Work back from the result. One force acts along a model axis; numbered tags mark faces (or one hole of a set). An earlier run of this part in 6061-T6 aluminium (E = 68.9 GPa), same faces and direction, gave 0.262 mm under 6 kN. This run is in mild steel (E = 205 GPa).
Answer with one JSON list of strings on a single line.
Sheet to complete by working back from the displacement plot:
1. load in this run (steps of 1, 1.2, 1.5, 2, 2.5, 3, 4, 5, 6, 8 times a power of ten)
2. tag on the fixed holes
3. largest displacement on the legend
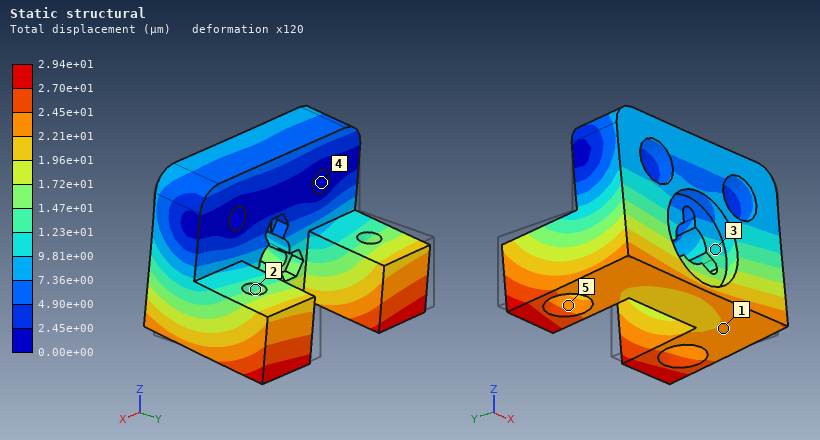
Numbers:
["2 kN", "4", "2.94e+01 µm"]
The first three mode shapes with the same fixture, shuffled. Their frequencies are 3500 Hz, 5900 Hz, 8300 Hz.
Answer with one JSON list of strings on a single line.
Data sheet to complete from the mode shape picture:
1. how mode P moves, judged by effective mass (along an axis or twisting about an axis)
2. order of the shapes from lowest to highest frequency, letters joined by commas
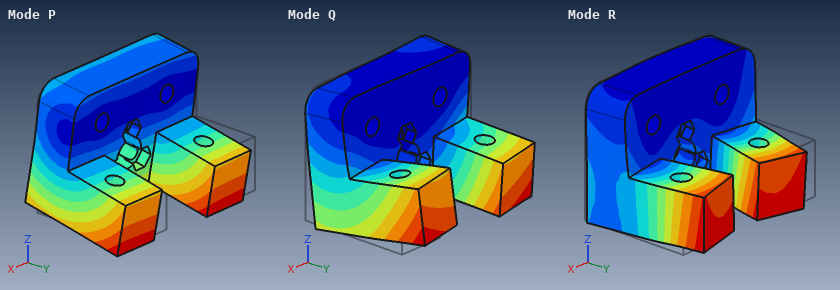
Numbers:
["along Y", "P, Q, R"]
